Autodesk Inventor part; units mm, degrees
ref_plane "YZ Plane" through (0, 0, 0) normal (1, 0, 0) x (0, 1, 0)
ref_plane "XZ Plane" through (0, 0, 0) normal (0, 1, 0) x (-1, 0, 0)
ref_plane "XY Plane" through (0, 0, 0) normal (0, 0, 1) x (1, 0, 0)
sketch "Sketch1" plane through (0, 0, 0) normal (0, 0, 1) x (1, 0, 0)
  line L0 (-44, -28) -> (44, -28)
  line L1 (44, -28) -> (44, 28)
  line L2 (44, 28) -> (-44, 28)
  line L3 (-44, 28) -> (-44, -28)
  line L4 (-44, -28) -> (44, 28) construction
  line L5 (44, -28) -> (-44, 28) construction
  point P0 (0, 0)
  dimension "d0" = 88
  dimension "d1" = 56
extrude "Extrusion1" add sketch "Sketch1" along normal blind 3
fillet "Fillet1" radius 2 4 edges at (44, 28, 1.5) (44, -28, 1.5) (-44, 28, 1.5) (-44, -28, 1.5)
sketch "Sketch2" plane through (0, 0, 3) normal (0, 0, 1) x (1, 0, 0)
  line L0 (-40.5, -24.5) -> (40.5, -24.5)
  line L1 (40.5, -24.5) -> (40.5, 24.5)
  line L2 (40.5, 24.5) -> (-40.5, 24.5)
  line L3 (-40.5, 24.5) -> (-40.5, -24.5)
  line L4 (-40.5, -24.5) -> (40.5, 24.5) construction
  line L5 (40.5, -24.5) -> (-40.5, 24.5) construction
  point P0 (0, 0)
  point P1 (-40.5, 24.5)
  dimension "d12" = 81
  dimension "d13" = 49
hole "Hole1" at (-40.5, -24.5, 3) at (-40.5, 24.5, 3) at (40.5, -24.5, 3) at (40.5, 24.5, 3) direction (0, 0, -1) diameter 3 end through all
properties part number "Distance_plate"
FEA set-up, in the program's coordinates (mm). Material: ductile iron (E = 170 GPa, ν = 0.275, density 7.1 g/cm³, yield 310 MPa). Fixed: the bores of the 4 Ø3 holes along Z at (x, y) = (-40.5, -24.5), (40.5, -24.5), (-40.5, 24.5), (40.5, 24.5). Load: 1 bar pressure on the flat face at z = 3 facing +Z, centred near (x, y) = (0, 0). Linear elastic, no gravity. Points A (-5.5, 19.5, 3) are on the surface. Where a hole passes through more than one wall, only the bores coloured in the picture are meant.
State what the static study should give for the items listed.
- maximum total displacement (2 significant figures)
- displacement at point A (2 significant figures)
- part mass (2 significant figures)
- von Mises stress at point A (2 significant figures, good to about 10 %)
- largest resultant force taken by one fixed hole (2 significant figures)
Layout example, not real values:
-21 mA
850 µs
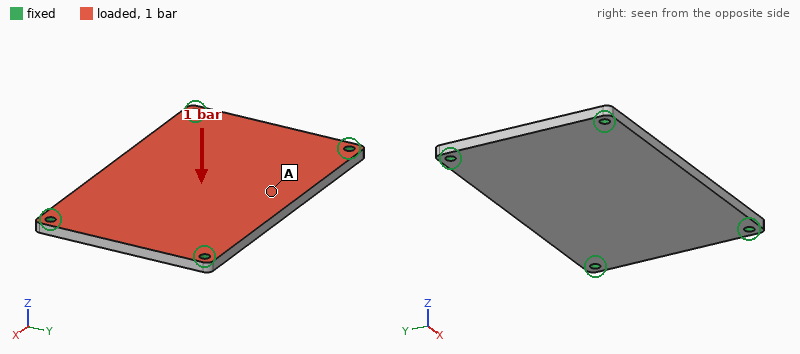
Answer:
47 µm
44 µm
100 g
22 MPa
120 N
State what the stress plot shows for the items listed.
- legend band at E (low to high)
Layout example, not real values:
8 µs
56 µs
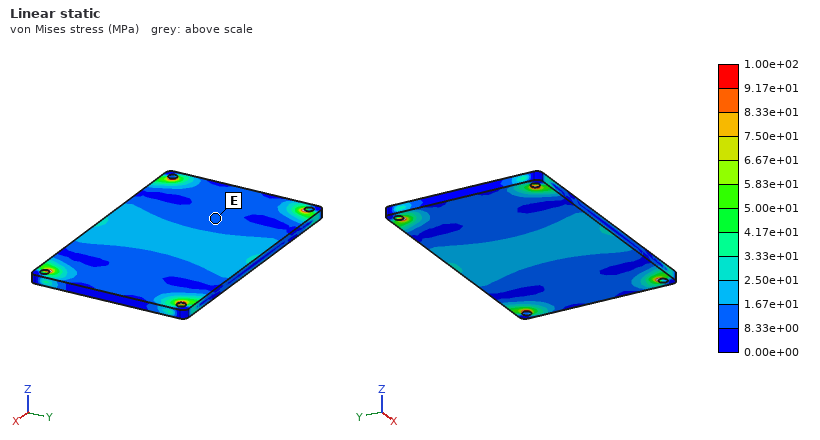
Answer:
8.33e+00 to 1.67e+01 MPa
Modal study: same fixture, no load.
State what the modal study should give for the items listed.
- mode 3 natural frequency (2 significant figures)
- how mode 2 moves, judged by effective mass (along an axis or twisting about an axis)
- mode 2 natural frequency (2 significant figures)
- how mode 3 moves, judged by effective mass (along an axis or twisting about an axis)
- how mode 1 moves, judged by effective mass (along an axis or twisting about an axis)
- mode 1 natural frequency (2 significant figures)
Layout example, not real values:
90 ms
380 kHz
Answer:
4700 Hz
twisting about X
3100 Hz
twisting about Y
along Z
1800 Hz
